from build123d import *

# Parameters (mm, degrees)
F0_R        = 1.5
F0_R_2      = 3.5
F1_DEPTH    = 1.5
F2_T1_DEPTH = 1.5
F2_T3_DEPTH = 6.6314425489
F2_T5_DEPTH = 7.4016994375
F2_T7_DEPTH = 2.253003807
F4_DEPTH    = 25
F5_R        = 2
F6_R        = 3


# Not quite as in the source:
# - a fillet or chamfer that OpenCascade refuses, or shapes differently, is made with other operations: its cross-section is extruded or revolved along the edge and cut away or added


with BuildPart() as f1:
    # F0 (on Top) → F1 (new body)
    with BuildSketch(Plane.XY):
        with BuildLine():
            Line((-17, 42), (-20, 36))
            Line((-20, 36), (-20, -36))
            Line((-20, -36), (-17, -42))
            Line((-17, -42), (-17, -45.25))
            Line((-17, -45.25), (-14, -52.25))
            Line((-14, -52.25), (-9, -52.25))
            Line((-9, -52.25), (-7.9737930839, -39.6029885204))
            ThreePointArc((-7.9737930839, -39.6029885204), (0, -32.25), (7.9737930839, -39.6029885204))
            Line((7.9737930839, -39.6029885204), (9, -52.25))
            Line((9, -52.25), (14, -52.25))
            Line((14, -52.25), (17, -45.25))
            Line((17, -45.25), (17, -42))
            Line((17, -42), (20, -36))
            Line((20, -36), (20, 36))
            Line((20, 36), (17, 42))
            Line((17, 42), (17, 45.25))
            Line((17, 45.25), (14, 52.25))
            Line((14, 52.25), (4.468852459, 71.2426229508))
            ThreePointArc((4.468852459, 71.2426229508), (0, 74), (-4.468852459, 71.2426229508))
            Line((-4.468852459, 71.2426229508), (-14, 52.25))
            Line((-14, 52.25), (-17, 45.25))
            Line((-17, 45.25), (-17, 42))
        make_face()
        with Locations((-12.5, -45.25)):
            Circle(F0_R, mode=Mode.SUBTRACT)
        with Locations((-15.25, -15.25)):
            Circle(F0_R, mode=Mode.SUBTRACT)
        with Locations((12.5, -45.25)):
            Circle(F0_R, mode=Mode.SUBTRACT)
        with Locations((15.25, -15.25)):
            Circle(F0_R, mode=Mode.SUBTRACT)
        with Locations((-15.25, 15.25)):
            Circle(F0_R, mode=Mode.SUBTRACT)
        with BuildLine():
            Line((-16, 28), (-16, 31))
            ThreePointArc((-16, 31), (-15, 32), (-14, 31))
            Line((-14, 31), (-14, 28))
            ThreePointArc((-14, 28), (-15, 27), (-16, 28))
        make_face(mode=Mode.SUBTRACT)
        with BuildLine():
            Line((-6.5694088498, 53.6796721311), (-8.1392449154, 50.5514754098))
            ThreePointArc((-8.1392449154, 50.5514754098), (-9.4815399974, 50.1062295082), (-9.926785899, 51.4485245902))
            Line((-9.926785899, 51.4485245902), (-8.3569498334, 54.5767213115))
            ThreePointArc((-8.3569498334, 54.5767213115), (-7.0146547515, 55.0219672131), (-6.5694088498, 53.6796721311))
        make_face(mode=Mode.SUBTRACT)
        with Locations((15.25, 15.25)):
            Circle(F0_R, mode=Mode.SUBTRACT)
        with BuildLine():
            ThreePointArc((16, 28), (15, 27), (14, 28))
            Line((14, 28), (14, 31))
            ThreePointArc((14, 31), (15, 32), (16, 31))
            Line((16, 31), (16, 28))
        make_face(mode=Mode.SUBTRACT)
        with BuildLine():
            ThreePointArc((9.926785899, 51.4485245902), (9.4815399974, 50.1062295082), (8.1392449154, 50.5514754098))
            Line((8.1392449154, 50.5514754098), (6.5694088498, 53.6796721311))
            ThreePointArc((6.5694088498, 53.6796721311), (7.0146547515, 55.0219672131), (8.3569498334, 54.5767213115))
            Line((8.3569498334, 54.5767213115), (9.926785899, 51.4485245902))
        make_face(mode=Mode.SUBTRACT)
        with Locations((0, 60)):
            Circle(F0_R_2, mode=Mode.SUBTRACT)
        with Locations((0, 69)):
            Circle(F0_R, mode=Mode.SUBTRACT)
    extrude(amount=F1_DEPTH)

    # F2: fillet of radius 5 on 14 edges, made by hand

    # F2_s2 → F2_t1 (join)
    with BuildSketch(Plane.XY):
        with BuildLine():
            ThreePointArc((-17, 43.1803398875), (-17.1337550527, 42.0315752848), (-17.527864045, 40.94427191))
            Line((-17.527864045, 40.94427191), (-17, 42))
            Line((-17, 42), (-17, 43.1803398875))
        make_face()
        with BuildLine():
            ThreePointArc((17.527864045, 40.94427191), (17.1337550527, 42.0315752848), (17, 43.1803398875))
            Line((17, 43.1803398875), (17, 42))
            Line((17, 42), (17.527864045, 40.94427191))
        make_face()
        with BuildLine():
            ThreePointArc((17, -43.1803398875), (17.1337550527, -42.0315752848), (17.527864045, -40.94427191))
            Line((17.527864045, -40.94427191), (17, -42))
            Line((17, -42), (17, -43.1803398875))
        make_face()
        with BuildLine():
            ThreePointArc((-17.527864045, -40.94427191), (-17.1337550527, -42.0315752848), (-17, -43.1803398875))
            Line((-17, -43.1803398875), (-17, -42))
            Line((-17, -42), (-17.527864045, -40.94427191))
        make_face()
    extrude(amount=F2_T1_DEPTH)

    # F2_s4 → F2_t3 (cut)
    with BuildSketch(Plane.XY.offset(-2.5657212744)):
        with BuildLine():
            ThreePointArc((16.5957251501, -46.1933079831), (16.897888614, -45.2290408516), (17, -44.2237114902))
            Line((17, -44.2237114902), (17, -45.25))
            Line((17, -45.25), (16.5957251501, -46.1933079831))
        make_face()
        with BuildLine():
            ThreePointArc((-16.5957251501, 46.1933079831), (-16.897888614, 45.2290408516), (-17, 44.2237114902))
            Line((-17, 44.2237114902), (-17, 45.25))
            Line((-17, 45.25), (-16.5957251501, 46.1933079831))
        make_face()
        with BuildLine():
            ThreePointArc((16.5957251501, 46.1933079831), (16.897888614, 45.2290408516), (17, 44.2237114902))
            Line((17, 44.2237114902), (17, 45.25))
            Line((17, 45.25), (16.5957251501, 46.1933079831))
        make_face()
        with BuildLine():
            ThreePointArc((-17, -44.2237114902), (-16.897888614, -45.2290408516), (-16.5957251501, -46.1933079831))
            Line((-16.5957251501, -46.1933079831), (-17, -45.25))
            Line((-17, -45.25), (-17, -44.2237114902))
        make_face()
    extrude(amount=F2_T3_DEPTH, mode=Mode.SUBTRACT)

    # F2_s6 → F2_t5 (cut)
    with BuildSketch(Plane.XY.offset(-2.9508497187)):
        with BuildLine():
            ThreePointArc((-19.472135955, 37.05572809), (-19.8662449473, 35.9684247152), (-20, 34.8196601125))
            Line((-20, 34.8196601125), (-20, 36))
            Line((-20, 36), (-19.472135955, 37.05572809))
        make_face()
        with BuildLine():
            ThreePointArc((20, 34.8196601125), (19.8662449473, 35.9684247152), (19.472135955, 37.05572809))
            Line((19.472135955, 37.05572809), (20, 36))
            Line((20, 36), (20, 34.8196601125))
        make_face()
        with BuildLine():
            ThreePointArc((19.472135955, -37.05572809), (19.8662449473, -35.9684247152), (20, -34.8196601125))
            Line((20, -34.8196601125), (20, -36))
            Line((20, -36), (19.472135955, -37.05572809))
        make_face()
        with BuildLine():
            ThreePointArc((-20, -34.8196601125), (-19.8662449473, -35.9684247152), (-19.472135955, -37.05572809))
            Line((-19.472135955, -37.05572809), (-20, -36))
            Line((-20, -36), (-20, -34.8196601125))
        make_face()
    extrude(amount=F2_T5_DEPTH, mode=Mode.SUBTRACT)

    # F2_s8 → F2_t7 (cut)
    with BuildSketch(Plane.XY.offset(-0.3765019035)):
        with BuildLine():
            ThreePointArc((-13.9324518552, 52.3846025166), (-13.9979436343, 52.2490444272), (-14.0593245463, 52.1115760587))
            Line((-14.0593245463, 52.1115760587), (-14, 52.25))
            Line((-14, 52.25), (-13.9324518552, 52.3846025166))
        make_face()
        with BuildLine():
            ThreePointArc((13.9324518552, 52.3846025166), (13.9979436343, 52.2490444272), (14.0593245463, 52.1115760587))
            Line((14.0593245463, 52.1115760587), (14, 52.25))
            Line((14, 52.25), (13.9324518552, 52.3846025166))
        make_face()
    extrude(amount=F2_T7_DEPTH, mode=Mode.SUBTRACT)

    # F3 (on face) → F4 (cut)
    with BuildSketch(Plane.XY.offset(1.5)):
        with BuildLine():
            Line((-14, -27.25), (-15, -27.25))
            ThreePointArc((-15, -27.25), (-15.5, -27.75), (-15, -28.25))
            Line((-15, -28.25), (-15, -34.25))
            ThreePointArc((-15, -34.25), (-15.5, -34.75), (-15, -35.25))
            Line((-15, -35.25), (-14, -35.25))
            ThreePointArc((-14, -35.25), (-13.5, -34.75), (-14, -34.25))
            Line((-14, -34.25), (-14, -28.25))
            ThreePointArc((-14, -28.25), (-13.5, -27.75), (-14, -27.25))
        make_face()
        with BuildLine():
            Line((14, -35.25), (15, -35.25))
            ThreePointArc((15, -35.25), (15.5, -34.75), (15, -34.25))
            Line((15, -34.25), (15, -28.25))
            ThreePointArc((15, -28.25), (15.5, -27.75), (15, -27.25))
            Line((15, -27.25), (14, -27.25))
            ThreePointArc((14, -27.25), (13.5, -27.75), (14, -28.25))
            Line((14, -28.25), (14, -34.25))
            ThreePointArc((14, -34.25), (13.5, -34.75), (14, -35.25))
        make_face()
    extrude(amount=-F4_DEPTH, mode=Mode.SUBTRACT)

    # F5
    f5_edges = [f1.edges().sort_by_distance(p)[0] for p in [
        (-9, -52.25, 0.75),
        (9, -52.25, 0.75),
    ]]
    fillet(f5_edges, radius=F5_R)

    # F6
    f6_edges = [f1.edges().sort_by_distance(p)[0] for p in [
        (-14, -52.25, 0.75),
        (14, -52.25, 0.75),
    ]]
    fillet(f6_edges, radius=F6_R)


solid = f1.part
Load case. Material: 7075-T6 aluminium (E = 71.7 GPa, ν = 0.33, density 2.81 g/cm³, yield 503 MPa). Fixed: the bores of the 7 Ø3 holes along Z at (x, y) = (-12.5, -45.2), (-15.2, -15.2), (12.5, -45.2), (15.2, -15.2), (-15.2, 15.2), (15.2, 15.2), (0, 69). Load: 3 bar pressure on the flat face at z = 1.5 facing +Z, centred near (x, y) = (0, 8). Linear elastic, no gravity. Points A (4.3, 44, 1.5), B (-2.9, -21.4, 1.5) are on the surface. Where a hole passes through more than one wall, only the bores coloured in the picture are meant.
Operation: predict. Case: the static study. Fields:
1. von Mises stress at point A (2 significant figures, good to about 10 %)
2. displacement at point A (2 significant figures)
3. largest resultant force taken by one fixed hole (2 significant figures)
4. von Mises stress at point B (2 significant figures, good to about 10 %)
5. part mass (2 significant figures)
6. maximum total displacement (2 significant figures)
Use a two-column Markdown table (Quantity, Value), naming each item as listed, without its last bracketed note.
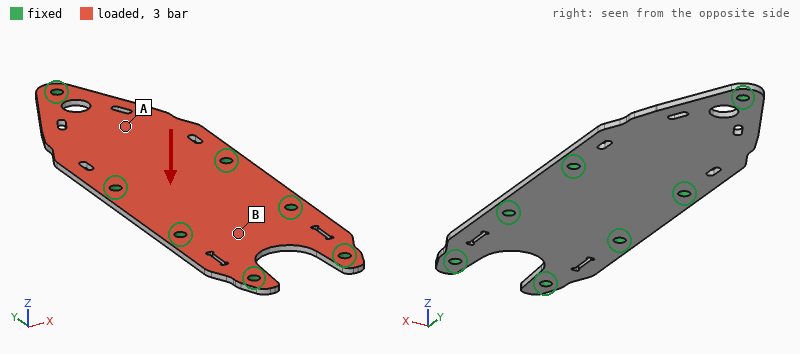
| Quantity | Value |
|---|---|
| von Mises stress at point A | 96 MPa |
| displacement at point A | 0.39 mm |
| largest resultant force taken by one fixed hole | 250 N |
| von Mises stress at point B | 27 MPa |
| part mass | 16 g |
| maximum total displacement | 0.44 mm |
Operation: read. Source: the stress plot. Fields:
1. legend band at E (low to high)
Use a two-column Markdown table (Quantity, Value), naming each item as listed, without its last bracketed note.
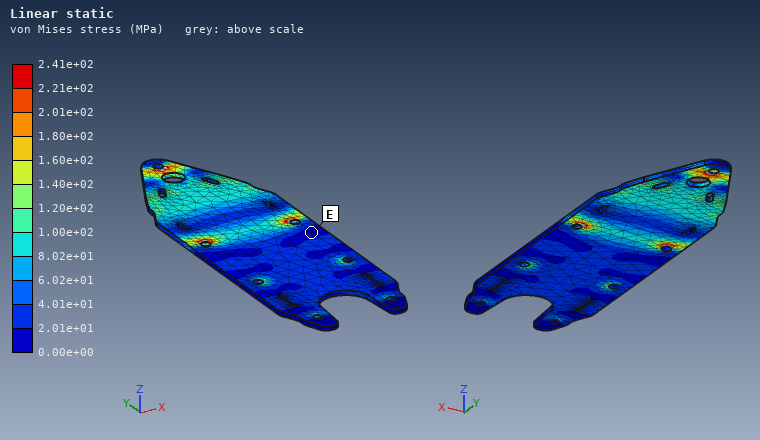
| Quantity | Value |
|---|---|
| legend band at E | 0.00e+00 to 2.01e+01 MPa |
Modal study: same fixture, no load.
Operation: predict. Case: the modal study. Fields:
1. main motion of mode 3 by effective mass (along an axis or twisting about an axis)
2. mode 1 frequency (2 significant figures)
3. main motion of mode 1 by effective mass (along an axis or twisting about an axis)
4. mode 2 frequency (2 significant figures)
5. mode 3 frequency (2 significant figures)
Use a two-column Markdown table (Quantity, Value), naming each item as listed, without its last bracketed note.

| Quantity | Value |
|---|---|
| main motion of mode 3 by effective mass | along Z |
| mode 1 frequency | 2400 Hz |
| main motion of mode 1 by effective mass | along Z |
| mode 2 frequency | 3100 Hz |
| mode 3 frequency | 6400 Hz |
